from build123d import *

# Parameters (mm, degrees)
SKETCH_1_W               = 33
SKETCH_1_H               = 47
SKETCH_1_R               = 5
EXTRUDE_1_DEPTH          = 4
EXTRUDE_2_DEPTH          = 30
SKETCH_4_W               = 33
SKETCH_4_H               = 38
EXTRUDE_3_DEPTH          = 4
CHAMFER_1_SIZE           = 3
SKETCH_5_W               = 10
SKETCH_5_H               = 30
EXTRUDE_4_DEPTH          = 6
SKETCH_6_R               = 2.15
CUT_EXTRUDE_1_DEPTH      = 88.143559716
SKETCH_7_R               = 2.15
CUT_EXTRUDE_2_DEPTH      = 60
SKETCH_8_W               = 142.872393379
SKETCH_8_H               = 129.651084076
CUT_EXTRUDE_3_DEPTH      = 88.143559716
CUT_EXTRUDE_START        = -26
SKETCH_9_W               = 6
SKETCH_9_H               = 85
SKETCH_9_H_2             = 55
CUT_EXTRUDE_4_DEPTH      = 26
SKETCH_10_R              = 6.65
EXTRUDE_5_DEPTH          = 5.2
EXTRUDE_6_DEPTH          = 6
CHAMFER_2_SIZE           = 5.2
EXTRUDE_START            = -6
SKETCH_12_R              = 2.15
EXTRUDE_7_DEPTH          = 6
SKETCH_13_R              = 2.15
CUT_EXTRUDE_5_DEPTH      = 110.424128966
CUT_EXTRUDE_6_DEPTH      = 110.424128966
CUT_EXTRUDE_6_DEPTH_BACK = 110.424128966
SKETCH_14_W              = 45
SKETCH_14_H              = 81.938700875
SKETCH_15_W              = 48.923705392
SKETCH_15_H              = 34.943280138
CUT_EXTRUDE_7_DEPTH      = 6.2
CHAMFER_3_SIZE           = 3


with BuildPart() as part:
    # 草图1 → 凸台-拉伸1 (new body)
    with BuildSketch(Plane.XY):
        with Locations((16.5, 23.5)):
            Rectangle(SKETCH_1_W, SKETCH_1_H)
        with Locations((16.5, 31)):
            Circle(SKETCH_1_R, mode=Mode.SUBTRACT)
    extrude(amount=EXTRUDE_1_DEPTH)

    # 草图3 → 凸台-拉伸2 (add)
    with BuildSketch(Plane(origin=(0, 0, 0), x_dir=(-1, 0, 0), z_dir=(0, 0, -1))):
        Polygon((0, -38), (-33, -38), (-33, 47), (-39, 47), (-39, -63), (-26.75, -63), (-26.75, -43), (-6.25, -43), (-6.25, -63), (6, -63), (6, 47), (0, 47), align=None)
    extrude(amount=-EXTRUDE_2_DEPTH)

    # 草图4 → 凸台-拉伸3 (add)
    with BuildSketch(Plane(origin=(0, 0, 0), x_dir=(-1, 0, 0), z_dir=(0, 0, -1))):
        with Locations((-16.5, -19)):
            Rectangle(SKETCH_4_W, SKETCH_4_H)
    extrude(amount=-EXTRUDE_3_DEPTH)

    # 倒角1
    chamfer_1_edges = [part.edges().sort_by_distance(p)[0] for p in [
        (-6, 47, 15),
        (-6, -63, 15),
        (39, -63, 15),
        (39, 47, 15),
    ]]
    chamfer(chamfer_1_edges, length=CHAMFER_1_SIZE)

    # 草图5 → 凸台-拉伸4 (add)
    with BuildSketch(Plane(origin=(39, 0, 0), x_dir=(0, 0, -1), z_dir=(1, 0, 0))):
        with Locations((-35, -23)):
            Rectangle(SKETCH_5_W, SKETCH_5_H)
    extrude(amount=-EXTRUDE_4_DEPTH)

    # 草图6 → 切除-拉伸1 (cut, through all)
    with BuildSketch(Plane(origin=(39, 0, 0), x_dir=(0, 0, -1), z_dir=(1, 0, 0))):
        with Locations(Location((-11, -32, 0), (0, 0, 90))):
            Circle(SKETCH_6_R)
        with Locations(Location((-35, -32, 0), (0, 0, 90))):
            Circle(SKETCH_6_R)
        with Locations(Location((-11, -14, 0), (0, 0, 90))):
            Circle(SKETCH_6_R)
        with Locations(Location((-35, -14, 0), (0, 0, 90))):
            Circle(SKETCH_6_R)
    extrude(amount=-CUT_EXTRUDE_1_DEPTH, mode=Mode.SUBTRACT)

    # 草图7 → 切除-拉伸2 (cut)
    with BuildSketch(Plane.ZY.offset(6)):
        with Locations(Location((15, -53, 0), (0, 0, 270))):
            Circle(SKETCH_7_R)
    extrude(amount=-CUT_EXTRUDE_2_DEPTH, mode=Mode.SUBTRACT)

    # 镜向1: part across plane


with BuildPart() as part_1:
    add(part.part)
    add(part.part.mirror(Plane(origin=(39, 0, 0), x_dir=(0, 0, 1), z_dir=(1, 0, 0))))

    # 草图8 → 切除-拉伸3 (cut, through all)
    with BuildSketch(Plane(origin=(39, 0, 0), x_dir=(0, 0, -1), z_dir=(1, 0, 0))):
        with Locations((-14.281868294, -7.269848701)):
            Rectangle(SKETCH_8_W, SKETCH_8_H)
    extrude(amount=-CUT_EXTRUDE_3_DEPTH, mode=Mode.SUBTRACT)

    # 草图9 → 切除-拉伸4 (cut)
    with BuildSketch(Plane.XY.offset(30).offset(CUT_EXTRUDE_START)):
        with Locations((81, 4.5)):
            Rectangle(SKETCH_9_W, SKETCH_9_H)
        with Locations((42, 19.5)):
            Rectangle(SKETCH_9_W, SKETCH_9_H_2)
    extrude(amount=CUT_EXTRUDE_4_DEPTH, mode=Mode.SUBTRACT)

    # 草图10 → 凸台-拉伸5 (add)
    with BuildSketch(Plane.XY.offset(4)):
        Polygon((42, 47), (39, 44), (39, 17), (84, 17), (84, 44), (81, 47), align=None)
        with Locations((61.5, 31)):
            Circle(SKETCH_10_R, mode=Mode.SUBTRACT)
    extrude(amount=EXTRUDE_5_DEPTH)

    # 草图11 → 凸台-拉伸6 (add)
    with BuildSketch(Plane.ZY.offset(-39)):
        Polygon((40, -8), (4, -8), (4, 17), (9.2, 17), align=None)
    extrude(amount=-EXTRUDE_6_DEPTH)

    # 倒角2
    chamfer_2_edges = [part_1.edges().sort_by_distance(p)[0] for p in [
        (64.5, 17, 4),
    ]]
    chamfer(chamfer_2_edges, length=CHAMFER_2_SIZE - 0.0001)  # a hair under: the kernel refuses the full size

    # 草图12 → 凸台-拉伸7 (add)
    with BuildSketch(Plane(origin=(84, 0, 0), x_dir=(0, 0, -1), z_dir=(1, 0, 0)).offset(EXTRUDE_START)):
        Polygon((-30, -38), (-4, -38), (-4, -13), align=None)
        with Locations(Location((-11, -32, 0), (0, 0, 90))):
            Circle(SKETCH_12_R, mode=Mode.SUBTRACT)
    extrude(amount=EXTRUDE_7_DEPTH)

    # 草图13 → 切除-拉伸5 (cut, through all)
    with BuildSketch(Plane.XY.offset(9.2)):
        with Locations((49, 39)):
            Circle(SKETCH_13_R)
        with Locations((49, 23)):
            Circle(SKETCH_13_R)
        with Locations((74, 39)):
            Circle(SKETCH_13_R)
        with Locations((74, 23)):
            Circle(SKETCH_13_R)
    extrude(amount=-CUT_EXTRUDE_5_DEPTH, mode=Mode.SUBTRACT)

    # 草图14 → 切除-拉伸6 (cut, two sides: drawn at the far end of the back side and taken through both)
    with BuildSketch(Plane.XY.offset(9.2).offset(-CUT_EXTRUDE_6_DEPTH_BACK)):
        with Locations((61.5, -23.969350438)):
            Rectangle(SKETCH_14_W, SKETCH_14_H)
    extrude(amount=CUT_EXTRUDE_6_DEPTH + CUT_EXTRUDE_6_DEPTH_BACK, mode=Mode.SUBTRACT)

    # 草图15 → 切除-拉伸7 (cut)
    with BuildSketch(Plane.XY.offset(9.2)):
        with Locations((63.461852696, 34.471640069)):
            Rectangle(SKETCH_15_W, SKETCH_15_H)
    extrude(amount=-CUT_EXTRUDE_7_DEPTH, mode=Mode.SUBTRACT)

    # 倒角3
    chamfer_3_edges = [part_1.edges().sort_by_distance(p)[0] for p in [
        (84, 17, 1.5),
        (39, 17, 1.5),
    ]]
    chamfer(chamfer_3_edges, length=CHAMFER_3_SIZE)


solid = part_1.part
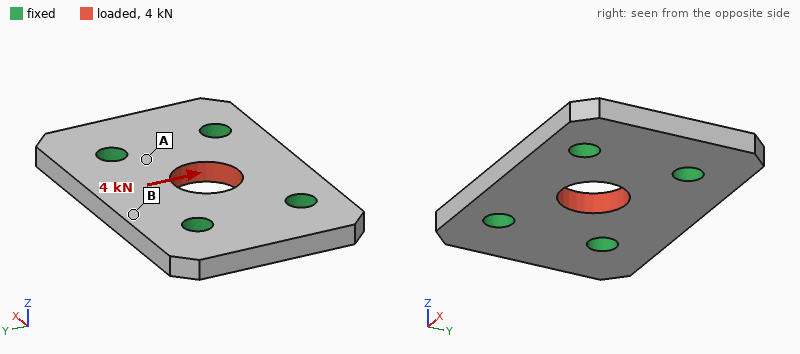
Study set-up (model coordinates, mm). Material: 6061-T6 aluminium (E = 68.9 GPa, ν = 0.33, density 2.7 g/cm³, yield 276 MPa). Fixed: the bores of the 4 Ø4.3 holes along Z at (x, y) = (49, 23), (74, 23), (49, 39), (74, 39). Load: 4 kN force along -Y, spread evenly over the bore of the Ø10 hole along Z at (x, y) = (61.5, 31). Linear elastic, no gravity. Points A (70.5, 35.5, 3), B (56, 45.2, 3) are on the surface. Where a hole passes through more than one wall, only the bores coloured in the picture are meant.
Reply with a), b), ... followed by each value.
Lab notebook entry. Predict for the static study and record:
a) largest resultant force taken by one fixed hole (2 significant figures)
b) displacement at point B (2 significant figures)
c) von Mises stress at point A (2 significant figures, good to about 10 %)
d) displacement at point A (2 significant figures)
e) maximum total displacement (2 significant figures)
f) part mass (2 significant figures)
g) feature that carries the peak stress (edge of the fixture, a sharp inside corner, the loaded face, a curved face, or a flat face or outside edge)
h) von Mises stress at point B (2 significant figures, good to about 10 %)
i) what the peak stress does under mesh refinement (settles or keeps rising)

a) 1.1 kN
b) 5.9 µm
c) 50 MPa
d) 2.8 µm
e) 12 µm
f) 9.7 g
g) edge of the fixture
h) 21 MPa
i) keeps rising
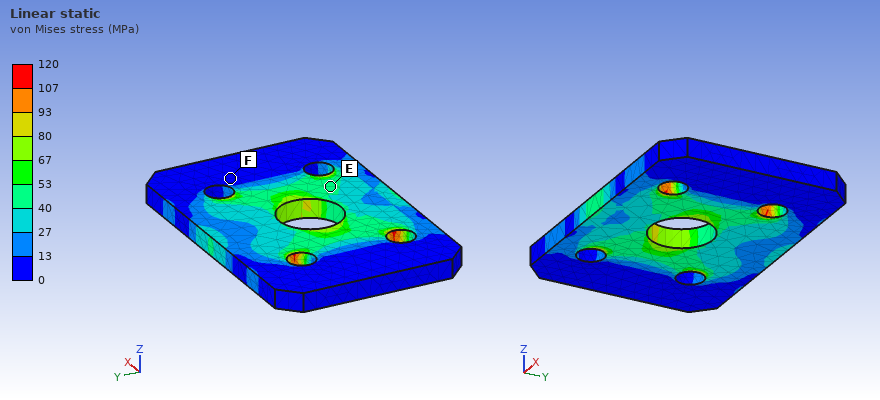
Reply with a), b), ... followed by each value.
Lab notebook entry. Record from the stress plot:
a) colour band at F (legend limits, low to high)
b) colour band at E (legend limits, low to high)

a) 0 to 13 MPa
b) 40 to 53 MPa
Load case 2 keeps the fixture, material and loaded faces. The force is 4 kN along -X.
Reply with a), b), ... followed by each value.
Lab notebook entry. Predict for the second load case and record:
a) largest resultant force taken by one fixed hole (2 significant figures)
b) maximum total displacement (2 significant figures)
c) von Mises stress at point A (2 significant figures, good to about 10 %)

a) 1.1 kN
b) 6.0 µm
c) 41 MPa
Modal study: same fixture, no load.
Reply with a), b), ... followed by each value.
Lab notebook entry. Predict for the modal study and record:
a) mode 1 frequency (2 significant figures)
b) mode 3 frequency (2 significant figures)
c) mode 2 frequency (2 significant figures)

a) 24 kHz
b) 28 kHz
c) 27 kHz
